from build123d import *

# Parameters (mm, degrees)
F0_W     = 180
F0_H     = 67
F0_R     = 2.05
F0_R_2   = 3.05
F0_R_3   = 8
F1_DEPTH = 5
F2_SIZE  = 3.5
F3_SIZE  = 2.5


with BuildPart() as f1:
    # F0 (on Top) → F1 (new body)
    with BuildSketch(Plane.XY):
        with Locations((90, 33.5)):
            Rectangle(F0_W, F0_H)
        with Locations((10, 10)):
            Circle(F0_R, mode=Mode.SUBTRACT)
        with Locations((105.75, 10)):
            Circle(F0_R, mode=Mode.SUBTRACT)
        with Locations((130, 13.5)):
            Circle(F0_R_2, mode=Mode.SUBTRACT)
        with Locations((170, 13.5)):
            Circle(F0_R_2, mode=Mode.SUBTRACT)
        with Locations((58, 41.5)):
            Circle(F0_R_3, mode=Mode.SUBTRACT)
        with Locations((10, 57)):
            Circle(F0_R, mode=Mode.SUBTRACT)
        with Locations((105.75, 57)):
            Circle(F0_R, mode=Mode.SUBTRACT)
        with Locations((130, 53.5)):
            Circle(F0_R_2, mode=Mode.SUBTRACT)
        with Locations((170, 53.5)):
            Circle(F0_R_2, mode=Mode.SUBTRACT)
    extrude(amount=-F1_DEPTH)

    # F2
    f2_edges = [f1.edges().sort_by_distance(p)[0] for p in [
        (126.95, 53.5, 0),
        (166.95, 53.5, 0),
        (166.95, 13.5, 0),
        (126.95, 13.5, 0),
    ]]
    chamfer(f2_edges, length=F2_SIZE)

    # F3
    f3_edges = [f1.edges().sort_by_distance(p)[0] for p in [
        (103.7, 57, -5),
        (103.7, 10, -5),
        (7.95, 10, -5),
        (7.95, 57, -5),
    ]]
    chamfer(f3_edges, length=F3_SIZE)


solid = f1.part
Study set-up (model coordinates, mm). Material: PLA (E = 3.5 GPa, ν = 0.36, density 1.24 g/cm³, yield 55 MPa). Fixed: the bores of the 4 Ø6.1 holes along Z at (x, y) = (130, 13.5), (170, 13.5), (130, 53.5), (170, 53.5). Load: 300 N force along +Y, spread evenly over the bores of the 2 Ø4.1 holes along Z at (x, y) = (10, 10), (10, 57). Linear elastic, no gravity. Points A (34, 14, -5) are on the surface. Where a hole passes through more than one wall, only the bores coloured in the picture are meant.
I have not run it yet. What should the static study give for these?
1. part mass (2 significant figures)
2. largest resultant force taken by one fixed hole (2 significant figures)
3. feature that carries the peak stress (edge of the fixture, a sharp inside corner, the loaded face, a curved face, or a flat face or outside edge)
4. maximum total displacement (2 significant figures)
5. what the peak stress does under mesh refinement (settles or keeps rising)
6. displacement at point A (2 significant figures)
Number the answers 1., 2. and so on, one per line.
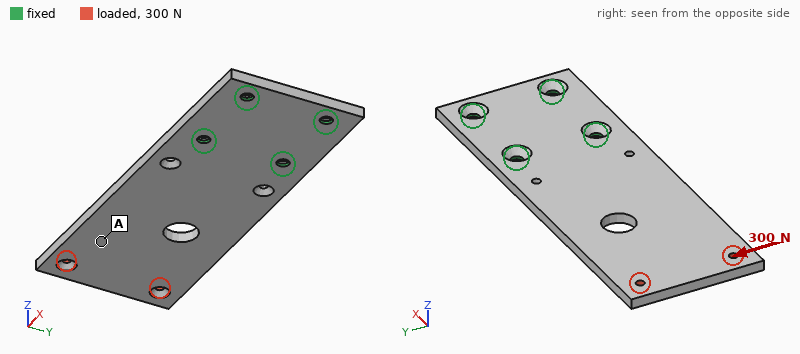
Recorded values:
1. 71 g
2. 630 N
3. edge of the fixture
4. 0.83 mm
5. keeps rising
6. 0.50 mm
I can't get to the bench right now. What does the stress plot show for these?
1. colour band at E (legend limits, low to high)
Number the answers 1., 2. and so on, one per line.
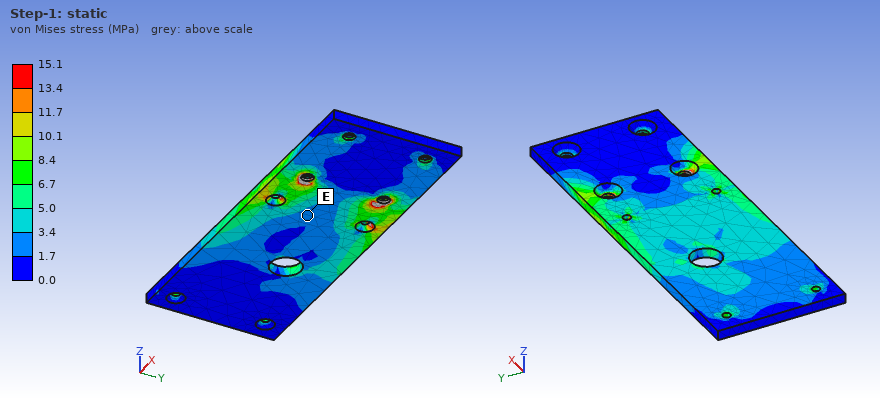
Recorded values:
1. 1.7 to 3.4 MPa
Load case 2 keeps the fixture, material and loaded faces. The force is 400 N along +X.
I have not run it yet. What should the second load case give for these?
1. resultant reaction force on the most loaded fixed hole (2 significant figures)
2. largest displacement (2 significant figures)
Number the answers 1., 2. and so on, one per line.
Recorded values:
1. 130 N
2. 2.2 mm
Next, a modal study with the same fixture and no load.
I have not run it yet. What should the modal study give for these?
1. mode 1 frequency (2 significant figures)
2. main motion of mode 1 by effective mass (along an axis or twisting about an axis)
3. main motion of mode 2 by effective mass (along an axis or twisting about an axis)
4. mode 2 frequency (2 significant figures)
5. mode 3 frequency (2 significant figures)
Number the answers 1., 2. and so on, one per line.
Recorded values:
1. 74 Hz
2. along Z
3. twisting about X
4. 310 Hz
5. 460 Hz
